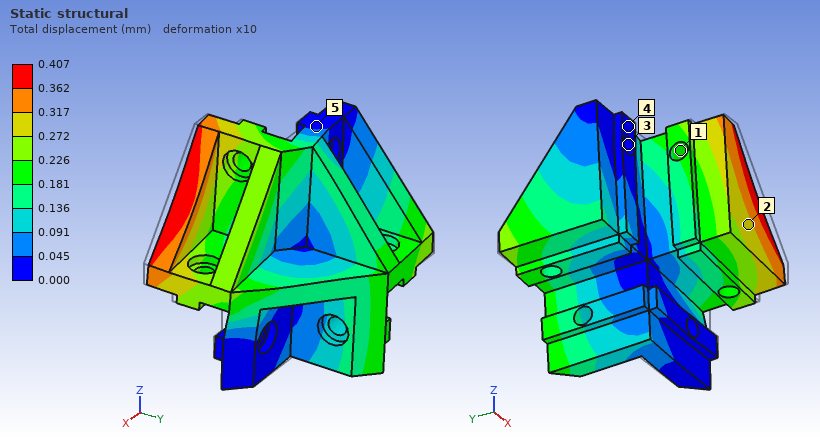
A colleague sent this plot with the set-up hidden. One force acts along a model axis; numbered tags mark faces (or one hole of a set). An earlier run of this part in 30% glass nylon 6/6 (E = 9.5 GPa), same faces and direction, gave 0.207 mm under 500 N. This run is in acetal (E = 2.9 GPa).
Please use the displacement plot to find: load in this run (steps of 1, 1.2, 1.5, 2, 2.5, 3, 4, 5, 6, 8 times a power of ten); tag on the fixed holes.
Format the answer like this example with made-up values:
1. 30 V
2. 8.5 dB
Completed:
1. 300 N
2. 3
